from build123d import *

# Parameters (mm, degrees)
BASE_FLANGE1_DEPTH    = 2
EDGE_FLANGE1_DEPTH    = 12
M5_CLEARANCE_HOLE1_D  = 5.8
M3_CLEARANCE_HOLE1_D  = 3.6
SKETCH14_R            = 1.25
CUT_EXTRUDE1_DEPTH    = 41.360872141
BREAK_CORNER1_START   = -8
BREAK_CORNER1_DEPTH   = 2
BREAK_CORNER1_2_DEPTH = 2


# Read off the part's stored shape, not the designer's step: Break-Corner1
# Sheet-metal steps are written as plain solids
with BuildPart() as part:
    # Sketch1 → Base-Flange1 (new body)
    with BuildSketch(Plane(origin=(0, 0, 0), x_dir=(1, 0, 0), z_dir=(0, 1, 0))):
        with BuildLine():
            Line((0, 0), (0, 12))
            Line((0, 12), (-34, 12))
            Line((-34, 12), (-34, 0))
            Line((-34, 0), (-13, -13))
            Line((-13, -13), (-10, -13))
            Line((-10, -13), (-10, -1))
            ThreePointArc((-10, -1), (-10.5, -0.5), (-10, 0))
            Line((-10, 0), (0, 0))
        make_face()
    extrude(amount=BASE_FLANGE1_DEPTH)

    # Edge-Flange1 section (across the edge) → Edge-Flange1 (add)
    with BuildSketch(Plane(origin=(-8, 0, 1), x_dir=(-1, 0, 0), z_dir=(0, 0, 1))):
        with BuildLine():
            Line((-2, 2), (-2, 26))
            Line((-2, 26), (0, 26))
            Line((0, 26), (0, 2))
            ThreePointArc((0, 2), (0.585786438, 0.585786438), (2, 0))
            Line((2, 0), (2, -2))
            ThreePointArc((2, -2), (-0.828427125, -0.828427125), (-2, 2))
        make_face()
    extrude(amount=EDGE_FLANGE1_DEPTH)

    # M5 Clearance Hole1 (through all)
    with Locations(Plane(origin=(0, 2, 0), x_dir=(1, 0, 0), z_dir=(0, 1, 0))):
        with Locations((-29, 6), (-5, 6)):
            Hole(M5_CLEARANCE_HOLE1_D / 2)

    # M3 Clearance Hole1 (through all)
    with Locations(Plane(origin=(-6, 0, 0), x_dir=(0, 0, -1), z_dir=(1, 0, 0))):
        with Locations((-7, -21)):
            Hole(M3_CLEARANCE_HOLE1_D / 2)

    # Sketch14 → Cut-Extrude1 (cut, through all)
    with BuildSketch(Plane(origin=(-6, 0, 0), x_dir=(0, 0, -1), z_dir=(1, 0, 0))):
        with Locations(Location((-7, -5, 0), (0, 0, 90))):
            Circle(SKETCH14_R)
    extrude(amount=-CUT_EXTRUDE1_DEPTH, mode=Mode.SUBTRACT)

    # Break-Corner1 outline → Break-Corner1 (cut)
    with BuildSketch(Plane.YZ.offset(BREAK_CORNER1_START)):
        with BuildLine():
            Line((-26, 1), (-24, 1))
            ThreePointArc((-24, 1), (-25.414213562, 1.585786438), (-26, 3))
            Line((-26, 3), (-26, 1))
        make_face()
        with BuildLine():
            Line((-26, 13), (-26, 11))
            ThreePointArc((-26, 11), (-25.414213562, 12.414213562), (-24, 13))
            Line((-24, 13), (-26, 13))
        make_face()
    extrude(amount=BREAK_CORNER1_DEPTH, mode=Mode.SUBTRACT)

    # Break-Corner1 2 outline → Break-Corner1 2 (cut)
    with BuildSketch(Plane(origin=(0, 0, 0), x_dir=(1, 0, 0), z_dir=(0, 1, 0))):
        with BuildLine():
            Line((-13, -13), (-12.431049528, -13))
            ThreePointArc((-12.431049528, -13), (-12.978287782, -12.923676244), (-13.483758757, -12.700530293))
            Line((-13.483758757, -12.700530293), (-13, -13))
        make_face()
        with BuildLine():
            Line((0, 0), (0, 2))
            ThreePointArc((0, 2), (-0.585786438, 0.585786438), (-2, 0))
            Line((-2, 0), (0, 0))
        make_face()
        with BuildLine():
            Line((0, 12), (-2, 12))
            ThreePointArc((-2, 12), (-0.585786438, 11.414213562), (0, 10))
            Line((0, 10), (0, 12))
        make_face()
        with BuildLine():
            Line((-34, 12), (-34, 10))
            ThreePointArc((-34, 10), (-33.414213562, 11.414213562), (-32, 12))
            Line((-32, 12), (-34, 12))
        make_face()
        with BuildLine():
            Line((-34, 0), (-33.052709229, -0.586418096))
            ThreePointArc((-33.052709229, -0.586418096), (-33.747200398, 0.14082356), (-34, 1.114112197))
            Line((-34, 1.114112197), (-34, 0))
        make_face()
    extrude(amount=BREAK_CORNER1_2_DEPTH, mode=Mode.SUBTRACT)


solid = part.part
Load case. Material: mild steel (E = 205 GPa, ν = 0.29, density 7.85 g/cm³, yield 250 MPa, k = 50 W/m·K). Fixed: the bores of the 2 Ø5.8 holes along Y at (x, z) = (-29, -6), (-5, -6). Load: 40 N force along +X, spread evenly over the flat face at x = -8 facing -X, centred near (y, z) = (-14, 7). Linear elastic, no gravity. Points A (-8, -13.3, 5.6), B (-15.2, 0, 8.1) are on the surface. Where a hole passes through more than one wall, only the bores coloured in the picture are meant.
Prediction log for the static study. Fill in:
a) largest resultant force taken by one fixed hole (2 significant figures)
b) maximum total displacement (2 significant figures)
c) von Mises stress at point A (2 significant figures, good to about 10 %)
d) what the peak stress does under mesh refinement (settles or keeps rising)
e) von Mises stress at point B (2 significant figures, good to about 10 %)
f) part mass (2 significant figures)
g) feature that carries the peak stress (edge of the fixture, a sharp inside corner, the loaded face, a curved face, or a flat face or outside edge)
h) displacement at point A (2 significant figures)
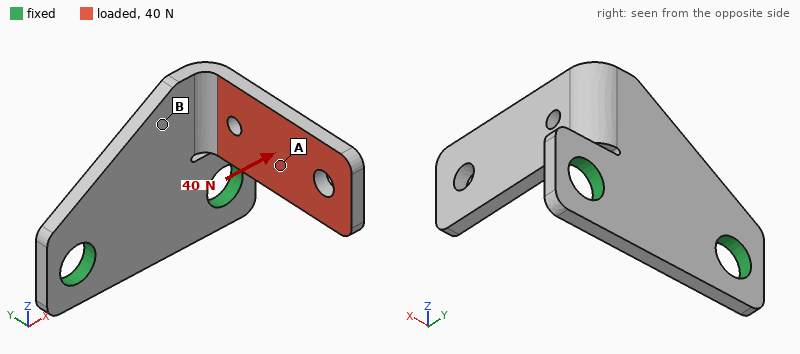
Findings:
48 N
0.16 mm
16 MPa
keeps rising
52 MPa
13 g
a sharp inside corner
0.072 mm
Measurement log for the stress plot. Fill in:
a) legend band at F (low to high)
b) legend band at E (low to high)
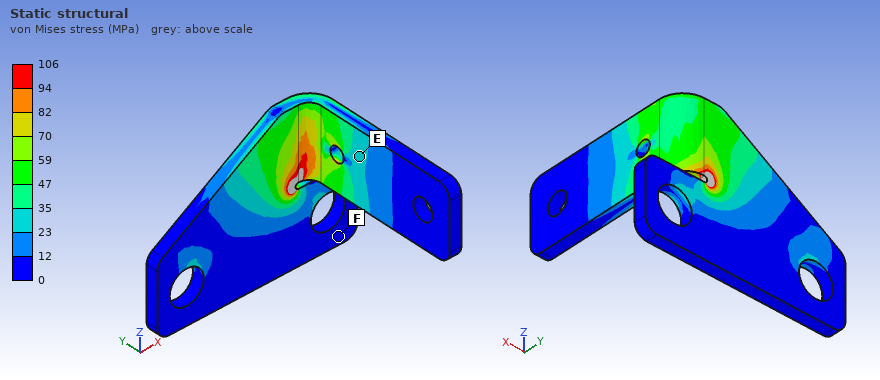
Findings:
0 to 12 MPa
23 to 35 MPa
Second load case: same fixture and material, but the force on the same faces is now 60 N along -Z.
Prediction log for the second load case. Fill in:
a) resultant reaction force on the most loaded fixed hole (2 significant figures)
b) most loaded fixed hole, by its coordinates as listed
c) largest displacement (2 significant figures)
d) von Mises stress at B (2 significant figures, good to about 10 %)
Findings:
56 N
(-5, -6)
0.18 mm
69 MPa
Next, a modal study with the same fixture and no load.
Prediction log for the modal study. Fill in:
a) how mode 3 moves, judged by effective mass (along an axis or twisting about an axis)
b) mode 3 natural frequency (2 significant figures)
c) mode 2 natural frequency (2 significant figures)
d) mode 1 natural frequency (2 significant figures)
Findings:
along Y
5800 Hz
1700 Hz
1400 Hz
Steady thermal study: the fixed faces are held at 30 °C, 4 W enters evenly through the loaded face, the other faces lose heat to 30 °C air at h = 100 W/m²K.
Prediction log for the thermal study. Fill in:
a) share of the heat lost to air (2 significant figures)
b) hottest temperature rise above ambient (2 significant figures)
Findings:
63 %
48 K
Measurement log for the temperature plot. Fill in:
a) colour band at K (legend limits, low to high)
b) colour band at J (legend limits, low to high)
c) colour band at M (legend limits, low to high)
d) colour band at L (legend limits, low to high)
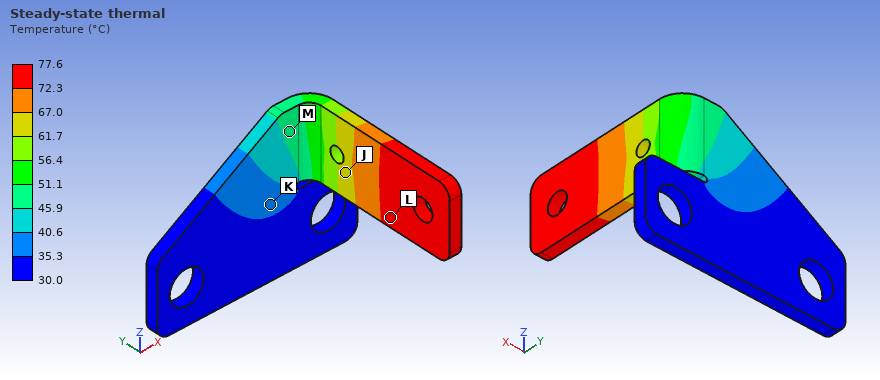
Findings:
35.3 to 40.6 °C
61.7 to 67.0 °C
45.9 to 51.1 °C
72.3 to 77.6 °C
